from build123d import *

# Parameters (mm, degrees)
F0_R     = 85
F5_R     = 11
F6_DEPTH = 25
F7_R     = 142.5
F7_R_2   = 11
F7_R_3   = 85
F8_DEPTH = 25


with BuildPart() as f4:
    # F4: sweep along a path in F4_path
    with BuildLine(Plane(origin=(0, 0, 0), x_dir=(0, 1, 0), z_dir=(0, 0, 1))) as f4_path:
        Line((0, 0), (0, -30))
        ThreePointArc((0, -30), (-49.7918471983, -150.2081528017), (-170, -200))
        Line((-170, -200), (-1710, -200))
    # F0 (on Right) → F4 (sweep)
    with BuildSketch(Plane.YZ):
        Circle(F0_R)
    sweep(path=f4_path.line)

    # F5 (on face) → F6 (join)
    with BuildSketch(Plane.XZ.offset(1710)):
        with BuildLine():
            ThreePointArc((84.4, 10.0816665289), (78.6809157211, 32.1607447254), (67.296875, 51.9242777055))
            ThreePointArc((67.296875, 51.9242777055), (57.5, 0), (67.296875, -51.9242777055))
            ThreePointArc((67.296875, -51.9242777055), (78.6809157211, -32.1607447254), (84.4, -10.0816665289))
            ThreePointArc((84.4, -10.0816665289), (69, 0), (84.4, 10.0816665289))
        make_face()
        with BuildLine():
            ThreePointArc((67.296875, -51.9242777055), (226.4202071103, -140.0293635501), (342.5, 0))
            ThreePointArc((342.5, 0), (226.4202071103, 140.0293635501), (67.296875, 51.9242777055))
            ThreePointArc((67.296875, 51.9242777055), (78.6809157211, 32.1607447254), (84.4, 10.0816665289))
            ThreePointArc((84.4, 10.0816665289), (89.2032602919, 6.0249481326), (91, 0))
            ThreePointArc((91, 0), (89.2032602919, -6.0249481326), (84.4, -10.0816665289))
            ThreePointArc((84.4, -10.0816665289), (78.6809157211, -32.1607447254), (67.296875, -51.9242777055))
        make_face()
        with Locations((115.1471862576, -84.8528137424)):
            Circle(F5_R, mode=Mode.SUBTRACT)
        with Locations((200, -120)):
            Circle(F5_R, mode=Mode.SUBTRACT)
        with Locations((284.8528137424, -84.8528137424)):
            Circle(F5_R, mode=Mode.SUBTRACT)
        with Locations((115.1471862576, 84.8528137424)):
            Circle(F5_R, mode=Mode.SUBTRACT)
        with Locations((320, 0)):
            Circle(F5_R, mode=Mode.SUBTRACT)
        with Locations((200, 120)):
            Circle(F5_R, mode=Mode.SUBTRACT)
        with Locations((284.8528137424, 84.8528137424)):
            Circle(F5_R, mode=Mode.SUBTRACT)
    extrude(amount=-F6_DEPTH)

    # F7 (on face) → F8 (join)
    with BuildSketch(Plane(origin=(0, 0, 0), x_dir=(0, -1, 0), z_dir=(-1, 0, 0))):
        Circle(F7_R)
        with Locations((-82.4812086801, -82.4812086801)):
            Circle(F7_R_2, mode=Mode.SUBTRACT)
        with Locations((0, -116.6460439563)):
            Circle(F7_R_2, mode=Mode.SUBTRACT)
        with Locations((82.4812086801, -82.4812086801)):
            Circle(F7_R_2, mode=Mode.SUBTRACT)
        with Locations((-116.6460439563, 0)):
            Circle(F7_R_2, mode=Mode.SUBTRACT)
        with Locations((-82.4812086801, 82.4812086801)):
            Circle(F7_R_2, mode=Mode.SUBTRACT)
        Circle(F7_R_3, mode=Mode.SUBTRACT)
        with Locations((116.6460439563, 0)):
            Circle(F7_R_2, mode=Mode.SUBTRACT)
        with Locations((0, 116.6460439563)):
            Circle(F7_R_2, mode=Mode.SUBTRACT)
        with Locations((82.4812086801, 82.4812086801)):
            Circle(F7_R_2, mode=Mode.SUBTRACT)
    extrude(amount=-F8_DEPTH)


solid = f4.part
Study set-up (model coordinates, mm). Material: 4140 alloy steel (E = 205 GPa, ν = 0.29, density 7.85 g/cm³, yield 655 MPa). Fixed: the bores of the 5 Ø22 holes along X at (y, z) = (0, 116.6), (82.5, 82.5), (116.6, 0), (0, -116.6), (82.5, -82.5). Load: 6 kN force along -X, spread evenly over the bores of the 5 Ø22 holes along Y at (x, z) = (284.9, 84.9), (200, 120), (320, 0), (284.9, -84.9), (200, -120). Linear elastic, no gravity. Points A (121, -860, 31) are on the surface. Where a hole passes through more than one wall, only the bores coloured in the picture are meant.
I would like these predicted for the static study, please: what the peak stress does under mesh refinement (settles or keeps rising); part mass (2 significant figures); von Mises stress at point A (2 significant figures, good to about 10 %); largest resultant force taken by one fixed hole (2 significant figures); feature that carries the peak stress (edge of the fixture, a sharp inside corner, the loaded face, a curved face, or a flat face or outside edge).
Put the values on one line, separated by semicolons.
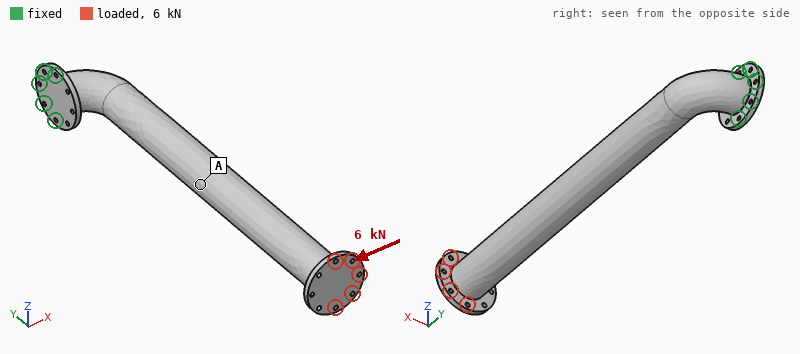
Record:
keeps rising; 340 kg; 9.7 MPa; 57 kN; edge of the fixture
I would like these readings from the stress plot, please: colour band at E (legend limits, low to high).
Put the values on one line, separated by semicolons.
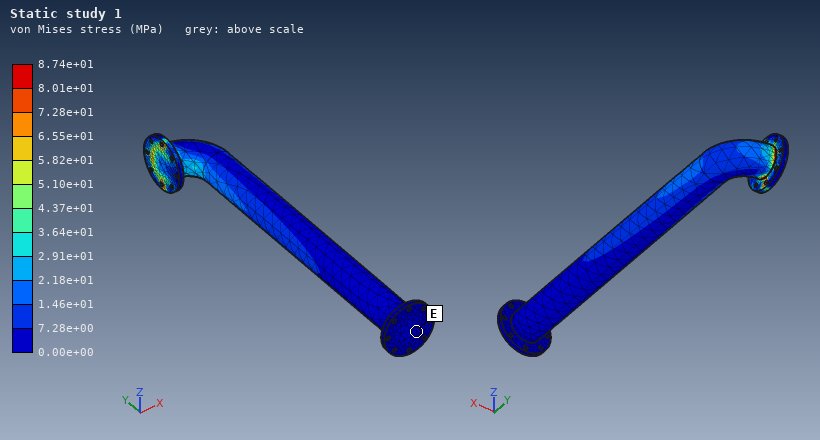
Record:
0.00e+00 to 7.28e+00 MPa
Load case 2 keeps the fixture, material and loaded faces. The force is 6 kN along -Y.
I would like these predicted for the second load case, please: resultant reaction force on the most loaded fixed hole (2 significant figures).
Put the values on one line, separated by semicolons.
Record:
8.0 kN
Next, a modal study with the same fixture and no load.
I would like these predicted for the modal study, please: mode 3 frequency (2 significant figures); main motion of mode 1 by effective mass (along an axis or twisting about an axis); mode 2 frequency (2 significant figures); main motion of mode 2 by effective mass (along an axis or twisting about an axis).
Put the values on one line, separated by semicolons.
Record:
160 Hz; along X; 33 Hz; along Z
